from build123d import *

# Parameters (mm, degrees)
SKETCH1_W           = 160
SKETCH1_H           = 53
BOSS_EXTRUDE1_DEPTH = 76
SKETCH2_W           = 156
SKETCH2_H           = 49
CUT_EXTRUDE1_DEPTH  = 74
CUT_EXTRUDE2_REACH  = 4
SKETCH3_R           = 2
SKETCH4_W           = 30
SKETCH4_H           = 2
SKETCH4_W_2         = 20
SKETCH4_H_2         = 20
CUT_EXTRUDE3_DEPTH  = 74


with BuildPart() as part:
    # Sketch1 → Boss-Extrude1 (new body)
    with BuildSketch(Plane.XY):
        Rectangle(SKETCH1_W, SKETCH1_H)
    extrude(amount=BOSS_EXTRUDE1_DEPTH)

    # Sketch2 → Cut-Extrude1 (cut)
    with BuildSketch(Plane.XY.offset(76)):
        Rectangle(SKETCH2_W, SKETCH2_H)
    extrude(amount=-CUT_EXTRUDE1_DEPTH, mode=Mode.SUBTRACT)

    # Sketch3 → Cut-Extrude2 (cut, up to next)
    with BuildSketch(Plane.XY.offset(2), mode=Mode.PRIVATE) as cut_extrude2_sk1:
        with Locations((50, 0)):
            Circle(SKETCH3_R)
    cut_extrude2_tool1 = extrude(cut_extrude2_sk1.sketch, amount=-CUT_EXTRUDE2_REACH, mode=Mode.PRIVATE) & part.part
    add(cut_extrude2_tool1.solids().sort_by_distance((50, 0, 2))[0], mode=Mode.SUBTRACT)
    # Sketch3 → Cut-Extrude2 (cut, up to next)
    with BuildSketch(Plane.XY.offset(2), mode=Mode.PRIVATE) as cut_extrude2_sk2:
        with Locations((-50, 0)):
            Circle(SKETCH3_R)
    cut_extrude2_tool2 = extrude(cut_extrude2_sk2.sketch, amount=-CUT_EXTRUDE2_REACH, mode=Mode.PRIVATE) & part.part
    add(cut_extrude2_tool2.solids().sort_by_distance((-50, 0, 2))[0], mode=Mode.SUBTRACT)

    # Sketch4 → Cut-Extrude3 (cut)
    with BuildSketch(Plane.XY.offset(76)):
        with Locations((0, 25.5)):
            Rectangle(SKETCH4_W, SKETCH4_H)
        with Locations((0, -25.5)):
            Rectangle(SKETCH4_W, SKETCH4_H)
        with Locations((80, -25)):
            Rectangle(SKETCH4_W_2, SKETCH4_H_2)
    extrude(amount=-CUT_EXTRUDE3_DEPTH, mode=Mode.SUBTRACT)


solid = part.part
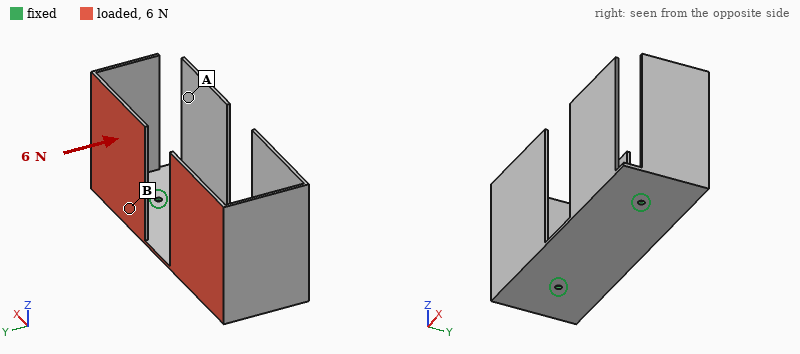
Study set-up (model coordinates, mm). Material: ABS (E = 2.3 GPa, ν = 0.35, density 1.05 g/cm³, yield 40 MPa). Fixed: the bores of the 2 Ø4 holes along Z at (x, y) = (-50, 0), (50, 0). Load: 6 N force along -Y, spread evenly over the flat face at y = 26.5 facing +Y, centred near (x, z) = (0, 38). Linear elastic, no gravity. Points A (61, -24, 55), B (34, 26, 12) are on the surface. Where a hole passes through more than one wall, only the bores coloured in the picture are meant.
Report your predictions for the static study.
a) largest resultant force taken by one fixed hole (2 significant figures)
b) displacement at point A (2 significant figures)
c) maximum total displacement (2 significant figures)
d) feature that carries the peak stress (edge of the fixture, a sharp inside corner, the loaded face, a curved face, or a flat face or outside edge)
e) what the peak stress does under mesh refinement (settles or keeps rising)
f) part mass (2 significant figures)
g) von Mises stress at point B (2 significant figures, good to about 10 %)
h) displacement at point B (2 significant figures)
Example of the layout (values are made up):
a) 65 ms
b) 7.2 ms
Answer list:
a) 3.0 N
b) 0.63 mm
c) 1.8 mm
d) edge of the fixture
e) keeps rising
f) 70 g
g) 0.62 MPa
h) 0.37 mm
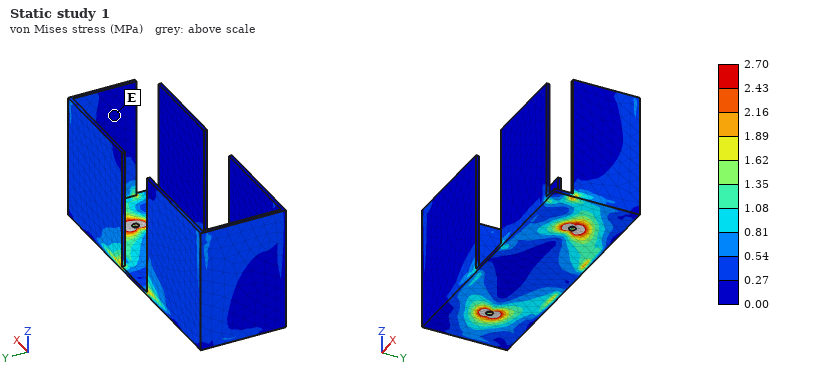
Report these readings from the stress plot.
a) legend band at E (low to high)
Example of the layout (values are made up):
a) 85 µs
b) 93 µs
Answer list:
a) 0.00 to 0.27 MPa
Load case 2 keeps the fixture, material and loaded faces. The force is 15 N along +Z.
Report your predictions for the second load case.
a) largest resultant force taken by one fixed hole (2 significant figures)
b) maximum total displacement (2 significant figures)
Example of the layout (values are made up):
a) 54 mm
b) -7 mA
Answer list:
a) 7.5 N
b) 1.8 mm
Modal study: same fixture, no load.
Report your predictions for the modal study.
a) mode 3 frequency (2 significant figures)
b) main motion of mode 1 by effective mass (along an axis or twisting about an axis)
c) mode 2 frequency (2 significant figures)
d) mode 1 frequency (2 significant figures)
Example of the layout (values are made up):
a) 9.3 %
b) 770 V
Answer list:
a) 71 Hz
b) along Y
c) 59 Hz
d) 54 Hz
